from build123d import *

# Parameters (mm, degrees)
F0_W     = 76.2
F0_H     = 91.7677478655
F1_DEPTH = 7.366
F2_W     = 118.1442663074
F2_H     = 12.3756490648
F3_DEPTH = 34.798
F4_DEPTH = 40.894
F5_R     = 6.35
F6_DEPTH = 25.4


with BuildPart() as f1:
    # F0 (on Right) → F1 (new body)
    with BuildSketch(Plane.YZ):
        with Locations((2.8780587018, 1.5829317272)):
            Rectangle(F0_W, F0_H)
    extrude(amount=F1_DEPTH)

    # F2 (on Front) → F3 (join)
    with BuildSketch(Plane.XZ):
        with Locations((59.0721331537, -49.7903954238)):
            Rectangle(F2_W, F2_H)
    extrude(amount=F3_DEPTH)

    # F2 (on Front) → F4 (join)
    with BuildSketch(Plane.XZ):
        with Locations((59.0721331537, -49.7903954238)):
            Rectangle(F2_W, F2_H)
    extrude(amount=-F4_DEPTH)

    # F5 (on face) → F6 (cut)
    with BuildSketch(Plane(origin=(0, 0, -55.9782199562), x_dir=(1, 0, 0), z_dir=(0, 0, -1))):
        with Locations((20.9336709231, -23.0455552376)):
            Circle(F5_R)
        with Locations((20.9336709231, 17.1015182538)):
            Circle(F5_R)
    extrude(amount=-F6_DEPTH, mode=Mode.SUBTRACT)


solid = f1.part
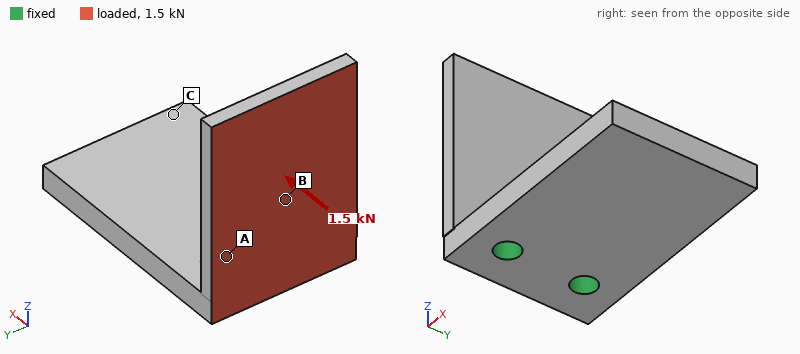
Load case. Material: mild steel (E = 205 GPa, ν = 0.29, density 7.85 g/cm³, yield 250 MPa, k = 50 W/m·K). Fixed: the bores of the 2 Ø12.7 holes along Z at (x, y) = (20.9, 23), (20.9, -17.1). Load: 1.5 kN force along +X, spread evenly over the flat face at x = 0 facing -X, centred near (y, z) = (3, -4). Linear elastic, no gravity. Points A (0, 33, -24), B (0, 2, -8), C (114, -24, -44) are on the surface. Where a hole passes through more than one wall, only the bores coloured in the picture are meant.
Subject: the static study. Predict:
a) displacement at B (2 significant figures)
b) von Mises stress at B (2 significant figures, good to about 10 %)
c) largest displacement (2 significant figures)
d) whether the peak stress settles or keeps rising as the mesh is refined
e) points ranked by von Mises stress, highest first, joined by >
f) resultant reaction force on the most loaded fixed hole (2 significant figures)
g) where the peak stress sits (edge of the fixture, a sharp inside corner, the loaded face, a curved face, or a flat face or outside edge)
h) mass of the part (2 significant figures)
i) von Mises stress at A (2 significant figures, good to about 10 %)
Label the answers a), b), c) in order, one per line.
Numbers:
a) 0.087 mm
b) 29 MPa
c) 0.30 mm
d) keeps rising
e) A > B > C
f) 770 N
g) a sharp inside corner
h) 1.2 kg
i) 53 MPa
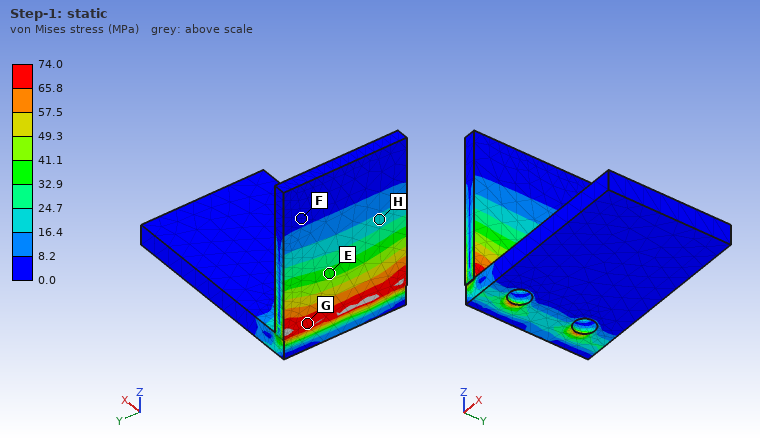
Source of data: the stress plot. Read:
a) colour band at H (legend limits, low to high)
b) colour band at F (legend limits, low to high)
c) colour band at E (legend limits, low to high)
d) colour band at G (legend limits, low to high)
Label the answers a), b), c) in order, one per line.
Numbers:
a) 16.4 to 24.7 MPa
b) 0.0 to 8.2 MPa
c) 32.9 to 41.1 MPa
d) 65.8 to 74.0 MPa
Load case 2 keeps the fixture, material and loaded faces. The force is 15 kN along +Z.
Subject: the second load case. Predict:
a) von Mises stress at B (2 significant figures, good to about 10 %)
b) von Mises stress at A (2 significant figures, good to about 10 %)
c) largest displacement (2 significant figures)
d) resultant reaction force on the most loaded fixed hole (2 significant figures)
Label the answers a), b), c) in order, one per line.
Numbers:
a) 53 MPa
b) 73 MPa
c) 0.39 mm
d) 7.5 kN
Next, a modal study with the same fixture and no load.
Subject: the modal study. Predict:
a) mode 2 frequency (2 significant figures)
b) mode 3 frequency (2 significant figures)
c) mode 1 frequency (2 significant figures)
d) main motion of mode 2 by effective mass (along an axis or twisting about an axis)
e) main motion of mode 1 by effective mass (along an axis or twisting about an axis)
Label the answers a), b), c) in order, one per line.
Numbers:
a) 1100 Hz
b) 1900 Hz
c) 650 Hz
d) along Z
e) along X
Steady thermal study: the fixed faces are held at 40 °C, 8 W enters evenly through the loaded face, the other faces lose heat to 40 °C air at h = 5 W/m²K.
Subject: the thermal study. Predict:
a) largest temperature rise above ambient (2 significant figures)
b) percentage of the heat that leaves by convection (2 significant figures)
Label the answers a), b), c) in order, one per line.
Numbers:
a) 14 K
b) 6.1 %
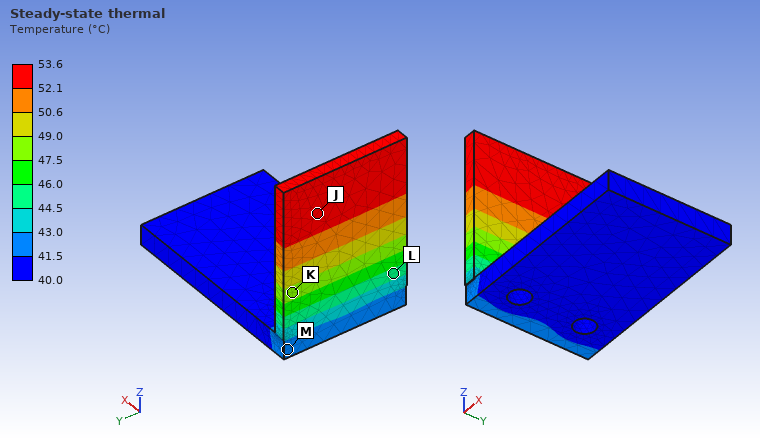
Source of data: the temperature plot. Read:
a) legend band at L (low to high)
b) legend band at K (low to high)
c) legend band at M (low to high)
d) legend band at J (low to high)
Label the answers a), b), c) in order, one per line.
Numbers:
a) 44.5 to 46.0 °C
b) 47.5 to 49.0 °C
c) 41.5 to 43.0 °C
d) 52.1 to 53.6 °C
